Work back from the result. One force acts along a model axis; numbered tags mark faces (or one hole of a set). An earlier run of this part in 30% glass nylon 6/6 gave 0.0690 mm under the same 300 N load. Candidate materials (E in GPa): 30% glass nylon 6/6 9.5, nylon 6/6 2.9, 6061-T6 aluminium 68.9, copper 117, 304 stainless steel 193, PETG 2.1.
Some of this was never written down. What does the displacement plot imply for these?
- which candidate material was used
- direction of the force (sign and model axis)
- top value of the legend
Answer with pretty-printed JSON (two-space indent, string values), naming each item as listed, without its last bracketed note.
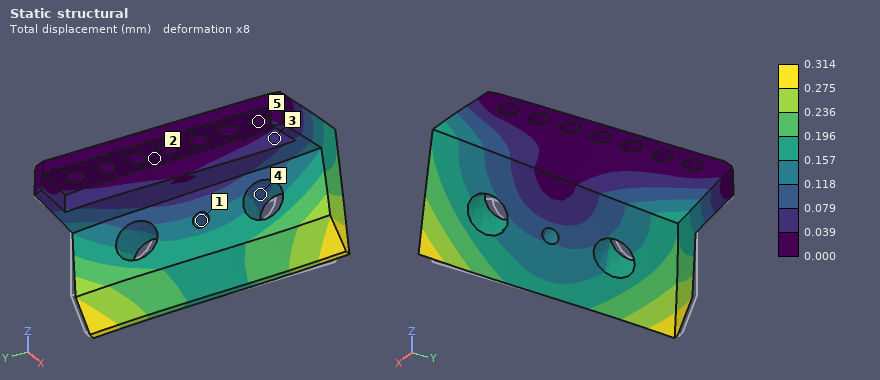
{
  "which candidate material was used": "PETG",
  "direction of the force": "-Y",
  "top value of the legend": "0.314 mm"
}
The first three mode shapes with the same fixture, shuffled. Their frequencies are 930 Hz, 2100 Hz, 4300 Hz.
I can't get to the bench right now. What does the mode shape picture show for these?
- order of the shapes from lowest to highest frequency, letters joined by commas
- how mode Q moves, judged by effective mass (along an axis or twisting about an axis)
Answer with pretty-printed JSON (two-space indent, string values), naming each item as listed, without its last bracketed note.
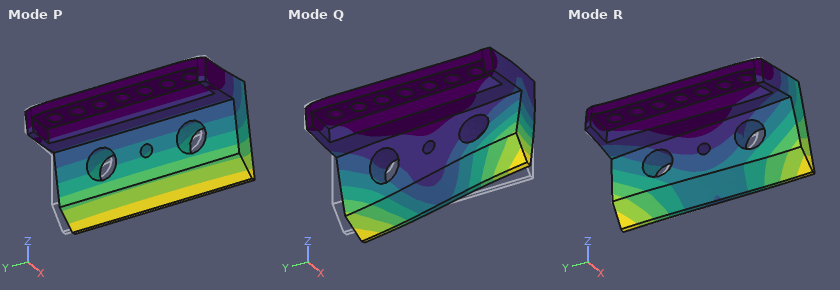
{
  "order of the shapes from lowest to highest frequency, letters joined by commas": "P, R, Q",
  "how mode Q moves, judged by effective mass": "along Y"
}
